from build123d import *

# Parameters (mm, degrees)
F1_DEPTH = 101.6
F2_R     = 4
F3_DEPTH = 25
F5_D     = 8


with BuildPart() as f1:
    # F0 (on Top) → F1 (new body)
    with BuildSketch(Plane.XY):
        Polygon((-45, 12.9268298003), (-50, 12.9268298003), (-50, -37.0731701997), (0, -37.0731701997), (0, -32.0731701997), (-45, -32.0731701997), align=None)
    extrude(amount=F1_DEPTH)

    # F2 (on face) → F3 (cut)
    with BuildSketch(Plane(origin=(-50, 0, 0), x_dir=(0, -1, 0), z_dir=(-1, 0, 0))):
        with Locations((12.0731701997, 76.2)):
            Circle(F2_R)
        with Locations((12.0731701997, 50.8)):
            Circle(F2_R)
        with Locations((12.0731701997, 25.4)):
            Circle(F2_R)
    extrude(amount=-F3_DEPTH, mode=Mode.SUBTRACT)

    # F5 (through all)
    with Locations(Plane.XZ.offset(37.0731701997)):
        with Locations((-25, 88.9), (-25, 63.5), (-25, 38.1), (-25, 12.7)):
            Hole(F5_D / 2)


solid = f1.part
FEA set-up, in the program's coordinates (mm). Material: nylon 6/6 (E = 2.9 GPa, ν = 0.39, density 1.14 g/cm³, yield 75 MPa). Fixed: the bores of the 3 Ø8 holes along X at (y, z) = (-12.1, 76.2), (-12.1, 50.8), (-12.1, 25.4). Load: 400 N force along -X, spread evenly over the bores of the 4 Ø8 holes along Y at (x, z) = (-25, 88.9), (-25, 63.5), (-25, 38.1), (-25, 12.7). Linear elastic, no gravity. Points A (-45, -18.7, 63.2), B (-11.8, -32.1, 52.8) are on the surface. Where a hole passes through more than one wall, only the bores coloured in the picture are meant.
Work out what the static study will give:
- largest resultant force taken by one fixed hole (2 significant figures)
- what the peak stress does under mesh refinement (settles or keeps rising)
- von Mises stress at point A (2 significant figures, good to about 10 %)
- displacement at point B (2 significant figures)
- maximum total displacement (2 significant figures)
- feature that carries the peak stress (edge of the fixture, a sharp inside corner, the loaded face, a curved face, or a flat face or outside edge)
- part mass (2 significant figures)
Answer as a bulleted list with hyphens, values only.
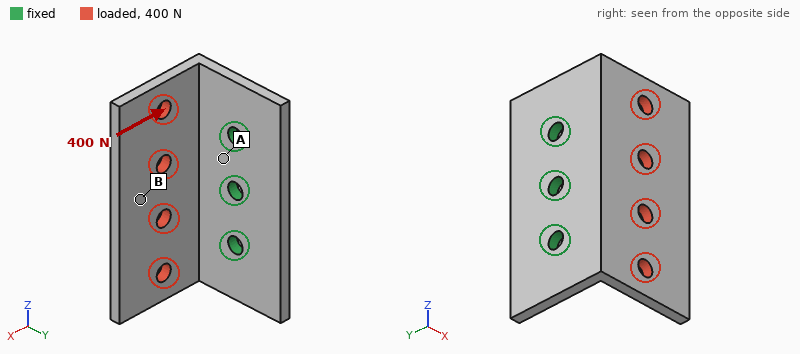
- 140 N
- keeps rising
- 11 MPa
- 1.1 mm
- 1.4 mm
- edge of the fixture
- 53 g
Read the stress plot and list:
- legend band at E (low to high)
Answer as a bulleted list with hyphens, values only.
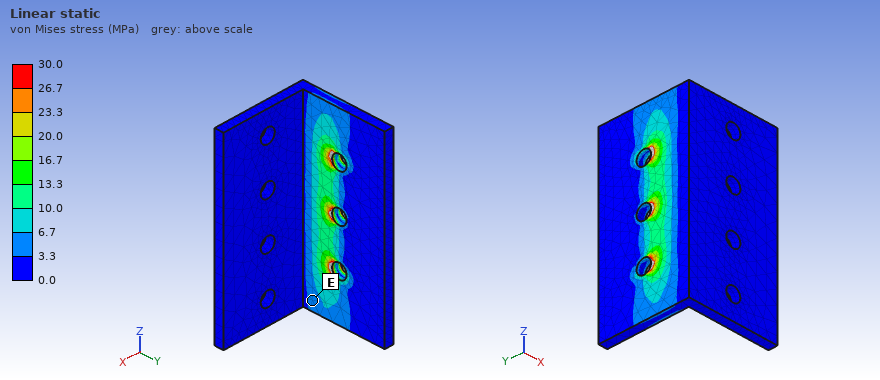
- 3.3 to 6.7 MPa
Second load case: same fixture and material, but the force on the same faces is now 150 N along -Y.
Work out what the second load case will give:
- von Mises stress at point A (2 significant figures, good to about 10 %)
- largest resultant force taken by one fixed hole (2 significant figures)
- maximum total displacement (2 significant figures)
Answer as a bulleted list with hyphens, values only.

- 6.5 MPa
- 58 N
- 1.4 mm
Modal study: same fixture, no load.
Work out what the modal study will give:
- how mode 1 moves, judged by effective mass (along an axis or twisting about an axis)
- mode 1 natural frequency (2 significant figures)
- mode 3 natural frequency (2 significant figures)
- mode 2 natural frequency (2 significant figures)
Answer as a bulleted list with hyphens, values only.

- along Y
- 350 Hz
- 940 Hz
- 560 Hz
